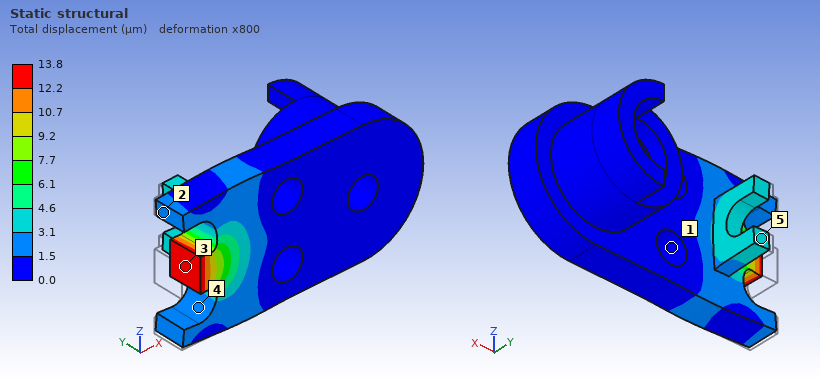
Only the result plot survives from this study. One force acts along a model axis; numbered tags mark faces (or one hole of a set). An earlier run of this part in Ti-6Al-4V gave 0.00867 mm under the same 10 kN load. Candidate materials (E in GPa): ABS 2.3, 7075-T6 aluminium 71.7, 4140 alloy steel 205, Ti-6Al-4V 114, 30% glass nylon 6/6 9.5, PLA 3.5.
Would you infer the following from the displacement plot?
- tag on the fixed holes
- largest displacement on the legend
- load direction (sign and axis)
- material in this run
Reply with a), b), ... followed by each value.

a) 1
b) 13.8 µm
c) +X
d) 7075-T6 aluminium
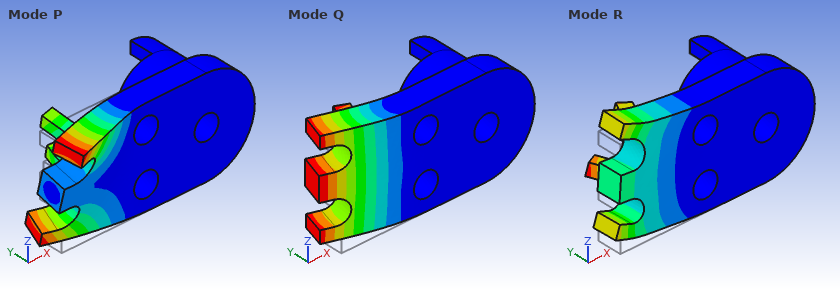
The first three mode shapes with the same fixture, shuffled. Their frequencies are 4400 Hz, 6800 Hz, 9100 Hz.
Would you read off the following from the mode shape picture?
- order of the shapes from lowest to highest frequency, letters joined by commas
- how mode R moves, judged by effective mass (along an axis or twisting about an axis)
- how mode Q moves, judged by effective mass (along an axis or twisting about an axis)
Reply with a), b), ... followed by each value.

a) Q, P, R
b) along Z
c) along Y
